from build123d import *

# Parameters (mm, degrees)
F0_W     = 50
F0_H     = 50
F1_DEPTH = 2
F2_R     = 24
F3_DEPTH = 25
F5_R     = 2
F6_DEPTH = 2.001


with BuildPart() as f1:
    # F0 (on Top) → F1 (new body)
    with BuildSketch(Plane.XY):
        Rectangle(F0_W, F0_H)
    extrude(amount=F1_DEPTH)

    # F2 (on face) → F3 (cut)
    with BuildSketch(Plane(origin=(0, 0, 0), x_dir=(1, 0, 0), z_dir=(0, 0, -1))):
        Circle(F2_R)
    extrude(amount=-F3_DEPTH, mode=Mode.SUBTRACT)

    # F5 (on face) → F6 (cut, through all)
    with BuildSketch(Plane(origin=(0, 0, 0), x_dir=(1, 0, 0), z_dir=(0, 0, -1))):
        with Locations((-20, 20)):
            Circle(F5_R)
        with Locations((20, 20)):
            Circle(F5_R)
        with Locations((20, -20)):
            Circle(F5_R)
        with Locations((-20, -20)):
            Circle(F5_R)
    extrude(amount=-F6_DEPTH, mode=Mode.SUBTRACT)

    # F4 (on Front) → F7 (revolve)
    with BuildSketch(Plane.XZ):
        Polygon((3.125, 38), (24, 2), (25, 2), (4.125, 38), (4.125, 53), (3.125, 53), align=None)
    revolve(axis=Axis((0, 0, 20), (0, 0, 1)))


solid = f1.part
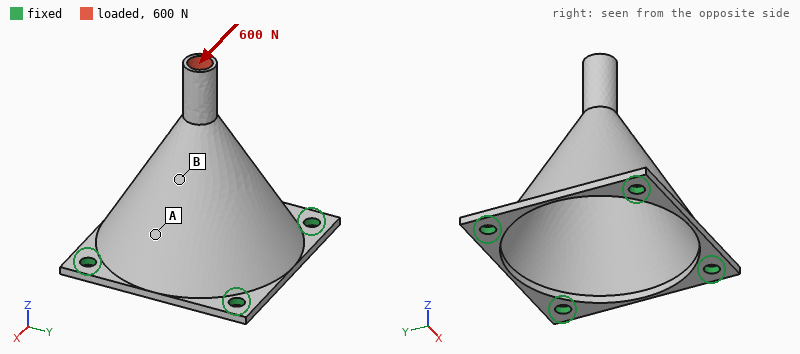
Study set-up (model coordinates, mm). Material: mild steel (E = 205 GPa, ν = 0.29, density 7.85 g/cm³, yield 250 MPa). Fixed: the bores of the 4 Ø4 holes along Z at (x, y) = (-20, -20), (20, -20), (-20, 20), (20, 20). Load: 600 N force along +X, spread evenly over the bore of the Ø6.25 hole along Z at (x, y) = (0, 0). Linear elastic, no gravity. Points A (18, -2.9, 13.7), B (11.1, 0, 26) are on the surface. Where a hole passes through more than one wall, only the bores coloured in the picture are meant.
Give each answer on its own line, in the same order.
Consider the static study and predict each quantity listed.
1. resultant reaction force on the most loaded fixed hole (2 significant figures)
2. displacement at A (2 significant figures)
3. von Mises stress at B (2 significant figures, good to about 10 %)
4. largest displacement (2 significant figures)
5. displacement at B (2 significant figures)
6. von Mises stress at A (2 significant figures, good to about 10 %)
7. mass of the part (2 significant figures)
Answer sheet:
430 N
8.1 µm
45 MPa
53 µm
11 µm
16 MPa
38 g
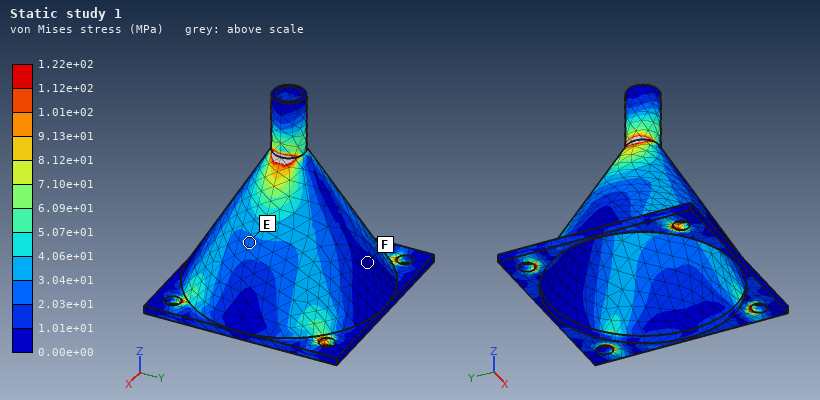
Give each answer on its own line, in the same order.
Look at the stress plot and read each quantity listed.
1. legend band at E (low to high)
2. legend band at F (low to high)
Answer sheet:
2.03e+01 to 3.04e+01 MPa
0.00e+00 to 1.01e+01 MPa
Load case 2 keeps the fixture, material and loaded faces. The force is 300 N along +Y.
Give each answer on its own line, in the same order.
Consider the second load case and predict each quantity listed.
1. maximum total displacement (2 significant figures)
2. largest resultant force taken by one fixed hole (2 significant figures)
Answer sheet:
27 µm
220 N
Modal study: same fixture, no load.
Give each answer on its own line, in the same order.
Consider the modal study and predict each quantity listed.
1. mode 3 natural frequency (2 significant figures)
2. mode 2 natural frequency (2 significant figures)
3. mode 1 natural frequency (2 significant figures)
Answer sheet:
11 kHz
9600 Hz
9600 Hz
